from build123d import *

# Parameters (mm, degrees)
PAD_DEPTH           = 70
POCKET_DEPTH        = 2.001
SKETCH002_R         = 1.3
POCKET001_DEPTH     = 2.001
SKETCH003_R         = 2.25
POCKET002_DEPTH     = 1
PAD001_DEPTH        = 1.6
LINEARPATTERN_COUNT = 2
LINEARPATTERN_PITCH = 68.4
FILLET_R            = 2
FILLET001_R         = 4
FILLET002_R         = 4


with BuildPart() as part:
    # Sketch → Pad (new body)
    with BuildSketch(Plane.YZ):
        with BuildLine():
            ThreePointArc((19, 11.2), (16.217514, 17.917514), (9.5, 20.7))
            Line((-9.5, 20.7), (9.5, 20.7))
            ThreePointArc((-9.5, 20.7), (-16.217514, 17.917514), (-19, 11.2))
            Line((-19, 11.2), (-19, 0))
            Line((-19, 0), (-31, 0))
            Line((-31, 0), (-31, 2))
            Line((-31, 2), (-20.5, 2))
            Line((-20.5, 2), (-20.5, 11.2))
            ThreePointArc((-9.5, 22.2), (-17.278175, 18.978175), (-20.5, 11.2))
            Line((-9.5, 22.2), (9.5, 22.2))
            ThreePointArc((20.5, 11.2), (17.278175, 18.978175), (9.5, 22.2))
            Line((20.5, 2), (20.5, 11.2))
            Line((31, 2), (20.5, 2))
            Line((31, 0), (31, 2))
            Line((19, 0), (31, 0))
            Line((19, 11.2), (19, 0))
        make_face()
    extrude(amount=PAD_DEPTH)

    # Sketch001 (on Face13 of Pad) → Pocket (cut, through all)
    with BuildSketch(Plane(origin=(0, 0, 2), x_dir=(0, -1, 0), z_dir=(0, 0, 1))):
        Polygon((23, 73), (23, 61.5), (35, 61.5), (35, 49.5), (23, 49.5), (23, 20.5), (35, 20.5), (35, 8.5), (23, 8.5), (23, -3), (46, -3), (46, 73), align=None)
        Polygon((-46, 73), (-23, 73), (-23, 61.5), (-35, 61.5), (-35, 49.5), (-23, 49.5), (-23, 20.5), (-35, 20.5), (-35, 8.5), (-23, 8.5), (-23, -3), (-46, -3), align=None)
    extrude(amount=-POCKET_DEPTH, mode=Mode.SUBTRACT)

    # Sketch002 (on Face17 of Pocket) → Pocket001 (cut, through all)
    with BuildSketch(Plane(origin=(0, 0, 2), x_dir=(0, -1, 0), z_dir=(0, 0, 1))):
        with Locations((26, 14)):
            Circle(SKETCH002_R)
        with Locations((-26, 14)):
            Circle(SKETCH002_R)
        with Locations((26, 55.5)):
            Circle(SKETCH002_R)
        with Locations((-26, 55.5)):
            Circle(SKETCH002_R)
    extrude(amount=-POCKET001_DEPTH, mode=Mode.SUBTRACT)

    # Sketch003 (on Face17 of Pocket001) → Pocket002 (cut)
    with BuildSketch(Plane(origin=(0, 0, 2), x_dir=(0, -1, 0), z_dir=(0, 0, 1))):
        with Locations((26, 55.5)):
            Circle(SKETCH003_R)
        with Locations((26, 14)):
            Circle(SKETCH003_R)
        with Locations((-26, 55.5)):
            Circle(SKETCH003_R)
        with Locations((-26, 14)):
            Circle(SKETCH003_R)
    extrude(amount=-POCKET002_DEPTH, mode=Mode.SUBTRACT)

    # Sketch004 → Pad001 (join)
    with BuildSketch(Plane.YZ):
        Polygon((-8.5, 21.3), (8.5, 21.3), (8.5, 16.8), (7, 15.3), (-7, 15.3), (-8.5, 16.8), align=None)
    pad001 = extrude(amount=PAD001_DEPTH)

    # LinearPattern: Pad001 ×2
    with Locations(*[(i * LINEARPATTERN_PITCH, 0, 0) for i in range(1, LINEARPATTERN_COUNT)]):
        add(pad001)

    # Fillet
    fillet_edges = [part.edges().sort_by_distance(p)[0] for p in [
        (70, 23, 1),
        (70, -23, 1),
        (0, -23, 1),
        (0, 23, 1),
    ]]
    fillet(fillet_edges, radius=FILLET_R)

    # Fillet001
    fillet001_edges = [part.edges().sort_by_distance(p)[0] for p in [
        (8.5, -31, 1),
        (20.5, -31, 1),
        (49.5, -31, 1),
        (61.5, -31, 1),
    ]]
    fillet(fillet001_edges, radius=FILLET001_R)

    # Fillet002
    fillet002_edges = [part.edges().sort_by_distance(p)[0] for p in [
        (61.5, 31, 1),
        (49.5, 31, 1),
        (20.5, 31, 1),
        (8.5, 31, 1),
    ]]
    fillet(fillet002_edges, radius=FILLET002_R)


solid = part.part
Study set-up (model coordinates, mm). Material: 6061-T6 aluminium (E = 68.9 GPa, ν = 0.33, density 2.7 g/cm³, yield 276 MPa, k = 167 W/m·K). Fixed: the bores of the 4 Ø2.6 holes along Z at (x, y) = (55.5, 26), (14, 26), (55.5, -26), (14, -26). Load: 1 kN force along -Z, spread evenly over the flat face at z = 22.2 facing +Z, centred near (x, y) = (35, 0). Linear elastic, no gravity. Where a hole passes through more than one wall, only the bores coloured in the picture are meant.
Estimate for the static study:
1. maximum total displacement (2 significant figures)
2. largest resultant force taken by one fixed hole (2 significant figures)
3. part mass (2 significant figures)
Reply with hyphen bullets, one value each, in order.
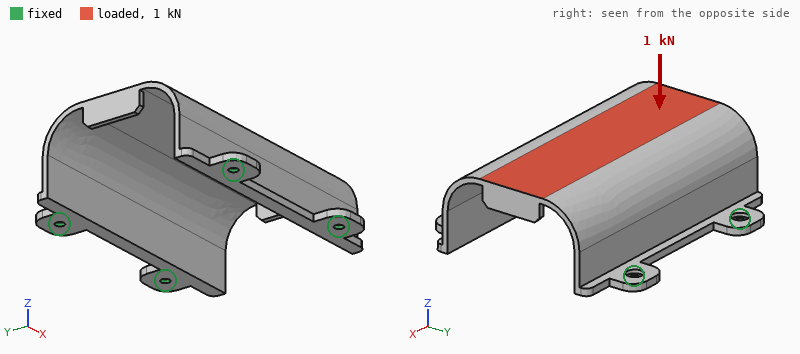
- 0.18 mm
- 300 N
- 25 g
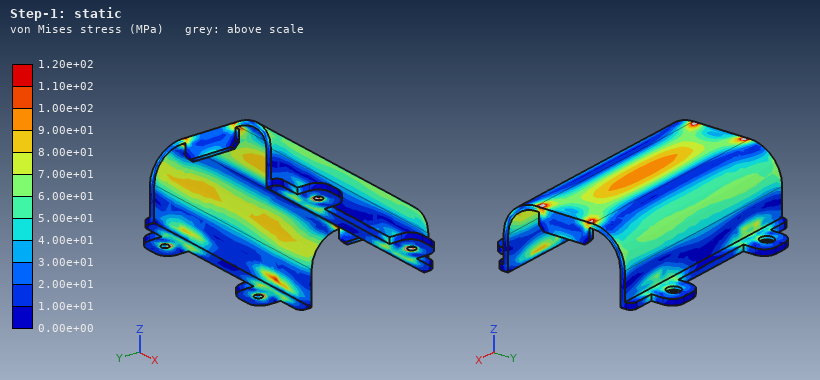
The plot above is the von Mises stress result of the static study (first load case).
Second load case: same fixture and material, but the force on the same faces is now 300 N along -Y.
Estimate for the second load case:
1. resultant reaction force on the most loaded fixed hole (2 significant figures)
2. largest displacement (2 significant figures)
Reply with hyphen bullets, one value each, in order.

- 93 N
- 0.17 mm
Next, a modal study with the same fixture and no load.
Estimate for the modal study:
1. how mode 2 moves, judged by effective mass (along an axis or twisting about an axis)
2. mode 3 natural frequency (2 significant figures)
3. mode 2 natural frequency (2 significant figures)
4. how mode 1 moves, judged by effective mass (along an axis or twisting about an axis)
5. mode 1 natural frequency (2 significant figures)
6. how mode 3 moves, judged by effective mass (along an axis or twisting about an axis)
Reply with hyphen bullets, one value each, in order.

- twisting about Z
- 4100 Hz
- 3400 Hz
- along Y
- 1800 Hz
- along X
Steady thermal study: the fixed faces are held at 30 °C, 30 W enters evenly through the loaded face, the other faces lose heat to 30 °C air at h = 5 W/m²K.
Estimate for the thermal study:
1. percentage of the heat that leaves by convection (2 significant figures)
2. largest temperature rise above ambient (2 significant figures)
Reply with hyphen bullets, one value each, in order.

- 5.0 %
- 42 K
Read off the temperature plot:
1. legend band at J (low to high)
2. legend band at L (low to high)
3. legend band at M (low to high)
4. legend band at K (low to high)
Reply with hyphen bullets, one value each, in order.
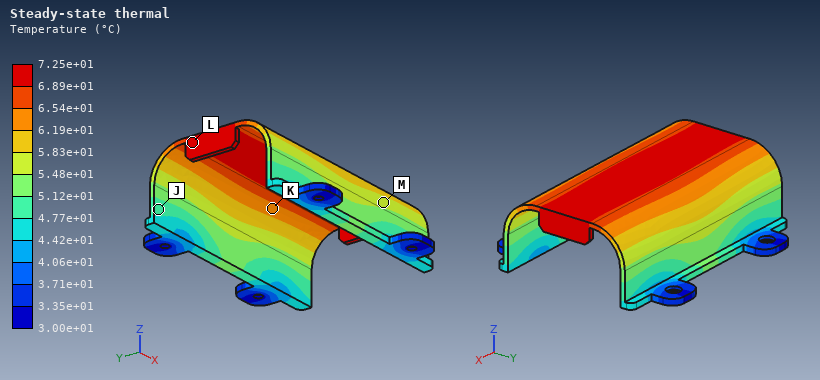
- 4.77e+01 to 5.12e+01 °C
- 6.89e+01 to 7.25e+01 °C
- 5.48e+01 to 5.83e+01 °C
- 6.19e+01 to 6.54e+01 °C
